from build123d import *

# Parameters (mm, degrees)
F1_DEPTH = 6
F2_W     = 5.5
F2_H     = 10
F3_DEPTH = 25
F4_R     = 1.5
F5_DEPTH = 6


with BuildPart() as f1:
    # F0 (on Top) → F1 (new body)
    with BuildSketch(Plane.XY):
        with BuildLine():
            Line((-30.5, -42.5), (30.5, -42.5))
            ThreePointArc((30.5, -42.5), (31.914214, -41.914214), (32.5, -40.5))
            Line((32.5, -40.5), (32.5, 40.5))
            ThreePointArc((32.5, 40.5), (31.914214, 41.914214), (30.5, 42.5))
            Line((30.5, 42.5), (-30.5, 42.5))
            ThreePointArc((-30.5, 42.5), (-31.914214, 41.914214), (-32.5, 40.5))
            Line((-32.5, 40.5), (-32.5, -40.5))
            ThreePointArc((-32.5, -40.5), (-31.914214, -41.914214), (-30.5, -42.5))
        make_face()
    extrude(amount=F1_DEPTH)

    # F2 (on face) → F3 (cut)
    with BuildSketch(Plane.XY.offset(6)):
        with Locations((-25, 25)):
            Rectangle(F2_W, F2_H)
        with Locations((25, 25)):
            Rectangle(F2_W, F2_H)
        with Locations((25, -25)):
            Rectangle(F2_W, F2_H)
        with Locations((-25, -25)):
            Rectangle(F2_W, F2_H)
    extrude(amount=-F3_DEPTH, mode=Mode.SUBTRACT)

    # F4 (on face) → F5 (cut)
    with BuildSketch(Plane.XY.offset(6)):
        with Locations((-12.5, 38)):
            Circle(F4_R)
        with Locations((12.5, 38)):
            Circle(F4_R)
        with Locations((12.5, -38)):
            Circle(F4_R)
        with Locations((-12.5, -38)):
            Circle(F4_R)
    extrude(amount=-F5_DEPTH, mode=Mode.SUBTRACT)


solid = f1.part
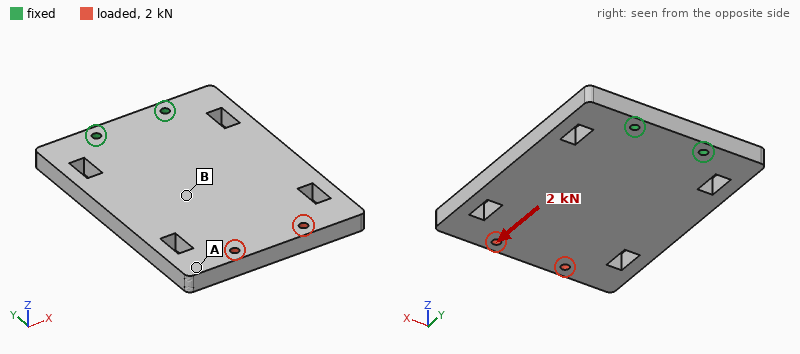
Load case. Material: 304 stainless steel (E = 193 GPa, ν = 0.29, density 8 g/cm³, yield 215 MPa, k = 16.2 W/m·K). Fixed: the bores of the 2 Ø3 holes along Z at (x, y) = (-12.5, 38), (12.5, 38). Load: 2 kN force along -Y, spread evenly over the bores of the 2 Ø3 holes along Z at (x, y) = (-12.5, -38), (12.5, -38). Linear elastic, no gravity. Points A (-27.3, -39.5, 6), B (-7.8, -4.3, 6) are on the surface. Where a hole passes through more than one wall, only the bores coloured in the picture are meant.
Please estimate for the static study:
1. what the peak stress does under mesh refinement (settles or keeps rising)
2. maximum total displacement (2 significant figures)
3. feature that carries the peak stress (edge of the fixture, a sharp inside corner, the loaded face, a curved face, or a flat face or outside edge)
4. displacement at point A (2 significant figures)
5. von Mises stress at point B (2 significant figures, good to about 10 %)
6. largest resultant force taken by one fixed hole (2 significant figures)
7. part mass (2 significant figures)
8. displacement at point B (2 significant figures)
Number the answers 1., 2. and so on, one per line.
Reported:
1. keeps rising
2. 3.7 µm
3. edge of the fixture
4. 2.3 µm
5. 7.0 MPa
6. 1.0 kN
7. 250 g
8. 1.8 µm
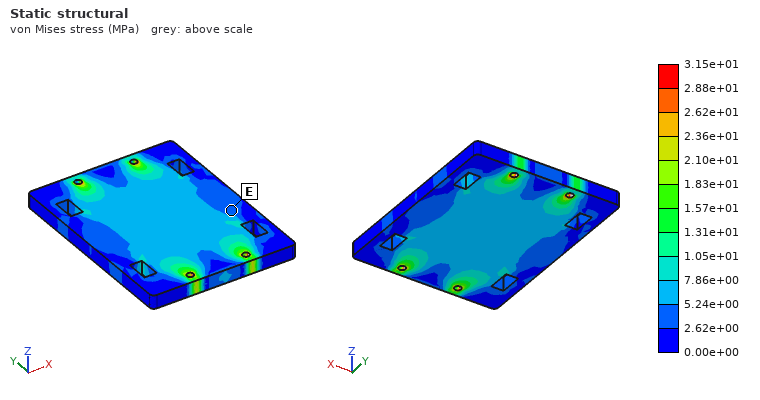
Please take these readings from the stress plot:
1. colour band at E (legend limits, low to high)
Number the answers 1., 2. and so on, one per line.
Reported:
1. 2.62e+00 to 5.24e+00 MPa
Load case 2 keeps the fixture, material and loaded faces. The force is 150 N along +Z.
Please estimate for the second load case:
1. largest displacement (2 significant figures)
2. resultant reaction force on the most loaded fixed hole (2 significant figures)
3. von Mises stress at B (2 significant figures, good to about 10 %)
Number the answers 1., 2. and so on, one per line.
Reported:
1. 0.14 mm
2. 75 N
3. 13 MPa
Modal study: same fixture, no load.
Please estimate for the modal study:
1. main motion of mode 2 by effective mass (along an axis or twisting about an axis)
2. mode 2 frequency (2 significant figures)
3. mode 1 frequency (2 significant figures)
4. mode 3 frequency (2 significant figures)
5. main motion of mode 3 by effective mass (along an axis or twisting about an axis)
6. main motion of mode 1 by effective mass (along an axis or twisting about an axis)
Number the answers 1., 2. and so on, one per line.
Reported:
1. twisting about Y
2. 1800 Hz
3. 640 Hz
4. 3200 Hz
5. along X
6. along Z
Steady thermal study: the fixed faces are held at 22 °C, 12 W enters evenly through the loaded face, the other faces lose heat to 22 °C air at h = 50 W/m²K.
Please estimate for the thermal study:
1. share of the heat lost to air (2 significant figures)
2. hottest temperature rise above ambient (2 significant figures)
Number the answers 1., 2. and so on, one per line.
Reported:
1. 91 %
2. 66 K
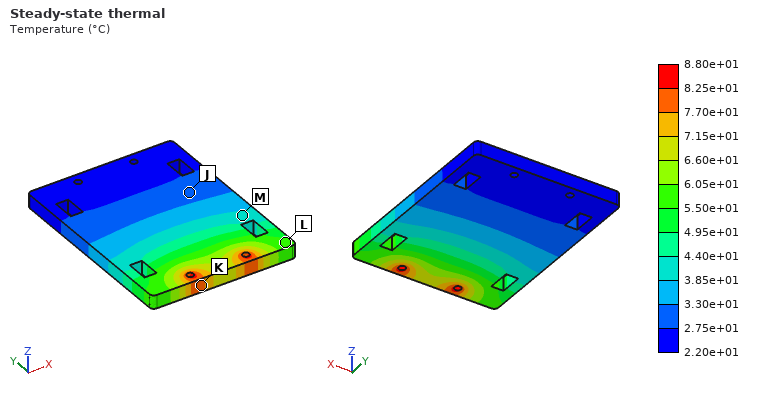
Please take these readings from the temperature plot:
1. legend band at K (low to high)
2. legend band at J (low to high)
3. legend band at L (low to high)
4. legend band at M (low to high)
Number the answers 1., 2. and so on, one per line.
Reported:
1. 7.70e+01 to 8.25e+01 °C
2. 2.75e+01 to 3.30e+01 °C
3. 5.50e+01 to 6.05e+01 °C
4. 3.85e+01 to 4.40e+01 °C
